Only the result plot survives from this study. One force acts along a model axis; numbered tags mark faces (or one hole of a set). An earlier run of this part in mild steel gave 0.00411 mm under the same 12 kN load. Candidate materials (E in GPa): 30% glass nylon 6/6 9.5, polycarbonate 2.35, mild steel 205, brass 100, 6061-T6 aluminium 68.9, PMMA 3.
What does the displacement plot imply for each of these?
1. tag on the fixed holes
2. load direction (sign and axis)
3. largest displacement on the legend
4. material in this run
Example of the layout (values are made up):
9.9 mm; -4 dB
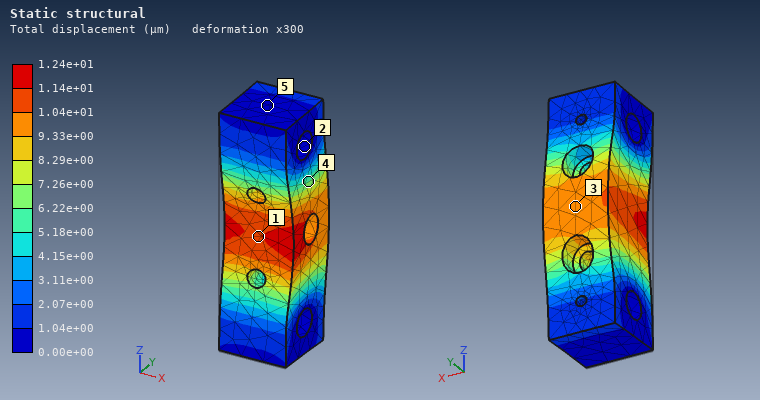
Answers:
2; +Y; 1.24e+01 µm; 6061-T6 aluminium
